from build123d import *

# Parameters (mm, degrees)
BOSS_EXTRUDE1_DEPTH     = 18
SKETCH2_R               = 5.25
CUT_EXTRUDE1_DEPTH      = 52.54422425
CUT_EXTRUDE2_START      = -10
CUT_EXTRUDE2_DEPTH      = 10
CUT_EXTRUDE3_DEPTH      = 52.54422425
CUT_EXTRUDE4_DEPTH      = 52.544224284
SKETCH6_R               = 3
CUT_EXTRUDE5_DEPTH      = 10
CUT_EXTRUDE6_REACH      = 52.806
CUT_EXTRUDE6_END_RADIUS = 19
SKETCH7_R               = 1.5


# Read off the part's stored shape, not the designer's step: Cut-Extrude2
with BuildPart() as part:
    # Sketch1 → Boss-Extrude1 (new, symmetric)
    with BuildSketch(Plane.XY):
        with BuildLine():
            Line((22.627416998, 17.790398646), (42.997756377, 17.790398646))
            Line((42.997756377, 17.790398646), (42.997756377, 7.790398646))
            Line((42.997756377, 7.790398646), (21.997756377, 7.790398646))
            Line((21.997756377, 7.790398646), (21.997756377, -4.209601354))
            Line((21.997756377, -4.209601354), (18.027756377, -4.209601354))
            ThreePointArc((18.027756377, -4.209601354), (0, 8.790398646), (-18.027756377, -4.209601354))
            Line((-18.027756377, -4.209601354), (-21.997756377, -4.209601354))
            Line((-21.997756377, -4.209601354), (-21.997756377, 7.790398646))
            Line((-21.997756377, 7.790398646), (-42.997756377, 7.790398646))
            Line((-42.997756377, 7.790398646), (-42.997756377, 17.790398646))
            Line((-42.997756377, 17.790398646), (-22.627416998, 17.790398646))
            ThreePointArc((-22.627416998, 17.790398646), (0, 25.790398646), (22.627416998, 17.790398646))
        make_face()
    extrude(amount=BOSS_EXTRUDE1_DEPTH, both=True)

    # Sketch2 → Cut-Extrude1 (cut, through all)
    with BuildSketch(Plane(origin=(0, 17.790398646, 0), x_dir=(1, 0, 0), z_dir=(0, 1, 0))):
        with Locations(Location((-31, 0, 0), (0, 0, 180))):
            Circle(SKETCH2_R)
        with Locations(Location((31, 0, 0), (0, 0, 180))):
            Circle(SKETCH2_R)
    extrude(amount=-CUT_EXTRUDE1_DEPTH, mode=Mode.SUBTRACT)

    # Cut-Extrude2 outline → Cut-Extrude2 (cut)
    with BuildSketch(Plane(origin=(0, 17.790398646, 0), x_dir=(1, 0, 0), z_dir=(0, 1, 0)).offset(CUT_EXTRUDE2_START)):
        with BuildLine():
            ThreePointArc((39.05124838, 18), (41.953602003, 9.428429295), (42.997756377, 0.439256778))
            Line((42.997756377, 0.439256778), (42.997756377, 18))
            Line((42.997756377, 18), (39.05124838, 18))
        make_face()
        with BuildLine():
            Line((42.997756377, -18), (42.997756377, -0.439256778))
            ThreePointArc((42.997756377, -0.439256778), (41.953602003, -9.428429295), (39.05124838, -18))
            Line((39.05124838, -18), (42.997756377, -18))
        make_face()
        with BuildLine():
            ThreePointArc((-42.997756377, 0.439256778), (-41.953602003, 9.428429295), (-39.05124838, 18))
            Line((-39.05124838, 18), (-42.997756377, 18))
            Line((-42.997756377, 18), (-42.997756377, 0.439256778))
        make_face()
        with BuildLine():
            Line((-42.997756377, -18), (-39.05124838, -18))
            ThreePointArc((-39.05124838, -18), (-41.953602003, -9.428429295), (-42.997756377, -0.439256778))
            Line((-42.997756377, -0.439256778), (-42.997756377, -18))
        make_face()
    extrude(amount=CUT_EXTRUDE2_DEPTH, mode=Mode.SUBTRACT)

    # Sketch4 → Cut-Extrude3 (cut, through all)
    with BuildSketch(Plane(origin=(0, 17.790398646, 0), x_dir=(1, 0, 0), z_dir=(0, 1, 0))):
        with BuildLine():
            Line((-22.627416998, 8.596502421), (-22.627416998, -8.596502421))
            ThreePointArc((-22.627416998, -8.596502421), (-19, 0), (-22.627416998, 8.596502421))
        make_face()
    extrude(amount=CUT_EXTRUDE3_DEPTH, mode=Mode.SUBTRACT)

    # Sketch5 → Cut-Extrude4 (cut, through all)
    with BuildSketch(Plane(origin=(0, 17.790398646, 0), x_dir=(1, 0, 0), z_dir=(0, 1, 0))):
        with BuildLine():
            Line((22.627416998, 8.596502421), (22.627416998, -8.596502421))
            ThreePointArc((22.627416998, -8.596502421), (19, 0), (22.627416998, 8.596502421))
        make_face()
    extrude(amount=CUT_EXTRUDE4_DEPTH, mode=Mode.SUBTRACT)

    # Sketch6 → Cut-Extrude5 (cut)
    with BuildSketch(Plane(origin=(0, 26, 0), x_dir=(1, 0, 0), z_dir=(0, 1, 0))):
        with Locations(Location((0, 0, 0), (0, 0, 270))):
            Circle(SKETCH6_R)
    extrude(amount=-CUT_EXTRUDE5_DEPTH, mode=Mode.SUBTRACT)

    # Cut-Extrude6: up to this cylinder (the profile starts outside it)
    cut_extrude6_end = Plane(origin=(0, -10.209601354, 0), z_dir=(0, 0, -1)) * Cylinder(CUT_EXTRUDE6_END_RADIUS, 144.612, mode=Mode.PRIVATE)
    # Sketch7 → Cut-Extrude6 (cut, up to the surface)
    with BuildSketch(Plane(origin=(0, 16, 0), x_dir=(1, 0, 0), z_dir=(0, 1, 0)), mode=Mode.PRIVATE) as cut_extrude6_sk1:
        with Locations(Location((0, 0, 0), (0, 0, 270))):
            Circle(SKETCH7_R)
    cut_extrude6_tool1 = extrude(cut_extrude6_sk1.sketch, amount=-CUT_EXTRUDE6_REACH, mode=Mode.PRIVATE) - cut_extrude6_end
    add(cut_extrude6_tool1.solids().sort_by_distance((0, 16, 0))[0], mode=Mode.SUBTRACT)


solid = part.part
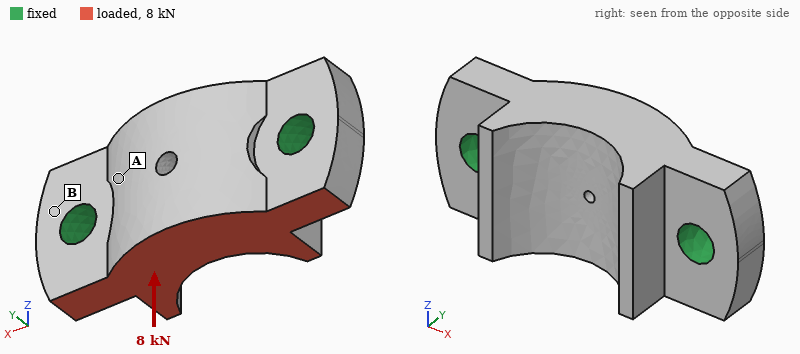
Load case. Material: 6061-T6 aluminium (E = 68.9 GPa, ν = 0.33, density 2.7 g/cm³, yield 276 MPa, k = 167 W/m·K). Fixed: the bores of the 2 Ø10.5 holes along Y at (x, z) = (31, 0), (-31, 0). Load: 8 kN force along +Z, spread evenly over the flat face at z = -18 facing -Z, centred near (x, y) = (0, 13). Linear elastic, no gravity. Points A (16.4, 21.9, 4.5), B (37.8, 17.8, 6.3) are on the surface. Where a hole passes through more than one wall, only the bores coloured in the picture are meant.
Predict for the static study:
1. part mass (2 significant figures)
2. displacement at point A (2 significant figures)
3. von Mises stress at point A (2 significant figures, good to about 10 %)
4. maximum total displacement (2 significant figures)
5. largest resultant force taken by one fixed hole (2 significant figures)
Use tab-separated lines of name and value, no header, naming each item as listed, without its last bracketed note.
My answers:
part mass	120 g
displacement at point A	6.6 µm
von Mises stress at point A	11 MPa
maximum total displacement	11 µm
largest resultant force taken by one fixed hole	4.0 kN
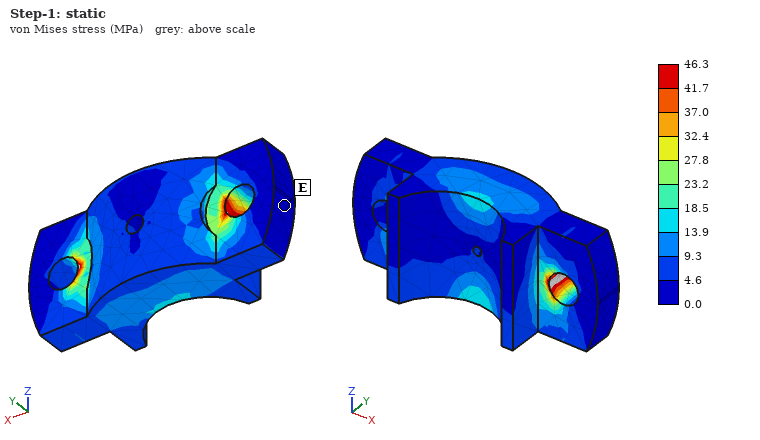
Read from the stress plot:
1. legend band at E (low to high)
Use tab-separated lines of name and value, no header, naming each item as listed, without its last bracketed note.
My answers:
legend band at E	0.0 to 4.6 MPa
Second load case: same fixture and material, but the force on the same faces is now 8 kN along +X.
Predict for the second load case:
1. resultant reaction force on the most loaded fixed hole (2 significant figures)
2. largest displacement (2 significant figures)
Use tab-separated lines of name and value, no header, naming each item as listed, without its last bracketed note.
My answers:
resultant reaction force on the most loaded fixed hole	4.5 kN
largest displacement	13 µm
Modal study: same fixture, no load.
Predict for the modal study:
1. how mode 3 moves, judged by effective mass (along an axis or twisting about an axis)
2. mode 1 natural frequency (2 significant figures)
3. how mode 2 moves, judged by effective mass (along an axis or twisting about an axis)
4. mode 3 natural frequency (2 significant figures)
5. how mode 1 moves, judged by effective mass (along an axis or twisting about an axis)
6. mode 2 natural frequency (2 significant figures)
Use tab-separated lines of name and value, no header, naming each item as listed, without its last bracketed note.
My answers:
how mode 3 moves, judged by effective mass	along Z
mode 1 natural frequency	11 kHz
how mode 2 moves, judged by effective mass	along Y
mode 3 natural frequency	16 kHz
how mode 1 moves, judged by effective mass	twisting about X
mode 2 natural frequency	12 kHz
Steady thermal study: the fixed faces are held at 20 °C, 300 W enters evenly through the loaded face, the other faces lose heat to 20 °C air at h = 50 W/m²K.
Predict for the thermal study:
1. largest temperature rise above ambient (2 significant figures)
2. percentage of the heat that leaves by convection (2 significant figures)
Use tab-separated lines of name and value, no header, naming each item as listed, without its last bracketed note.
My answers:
largest temperature rise above ambient	49 K
percentage of the heat that leaves by convection	3.0 %
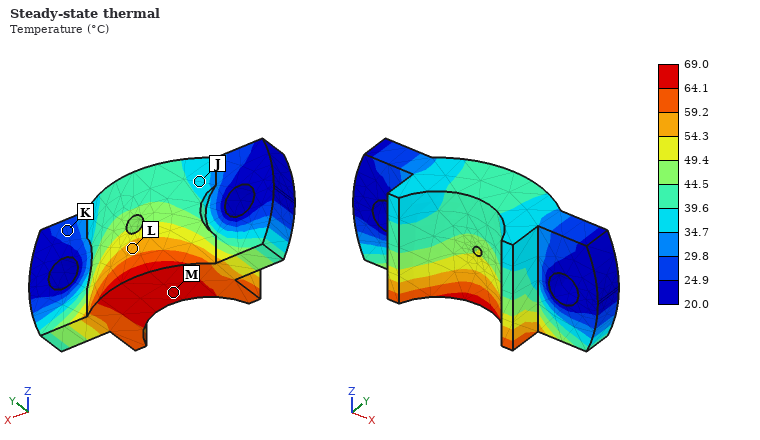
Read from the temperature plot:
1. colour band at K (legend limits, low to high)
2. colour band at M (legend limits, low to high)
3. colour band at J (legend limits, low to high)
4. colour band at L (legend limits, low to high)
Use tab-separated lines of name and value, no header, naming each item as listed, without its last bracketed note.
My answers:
colour band at K	24.9 to 29.8 °C
colour band at M	64.1 to 69.0 °C
colour band at J	34.7 to 39.6 °C
colour band at L	54.3 to 59.2 °C
